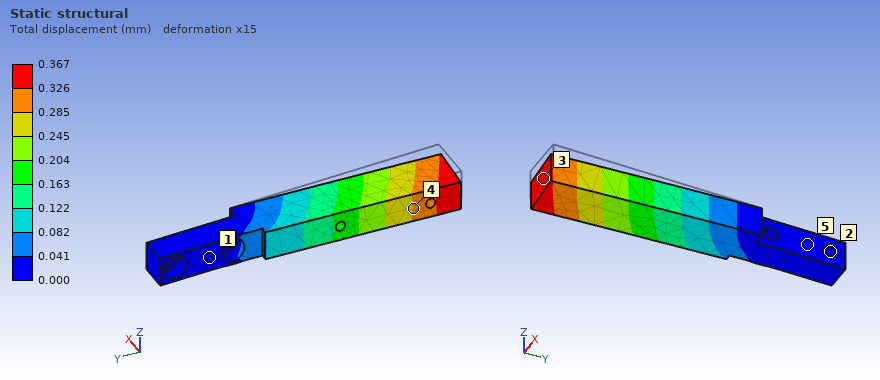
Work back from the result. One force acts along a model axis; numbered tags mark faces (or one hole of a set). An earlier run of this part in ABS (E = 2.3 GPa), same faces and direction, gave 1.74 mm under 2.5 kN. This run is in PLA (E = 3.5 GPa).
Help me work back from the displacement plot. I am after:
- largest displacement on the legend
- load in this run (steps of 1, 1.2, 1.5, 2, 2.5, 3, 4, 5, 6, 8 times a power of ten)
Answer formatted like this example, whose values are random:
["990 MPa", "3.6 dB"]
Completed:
["0.367 mm", "800 N"]
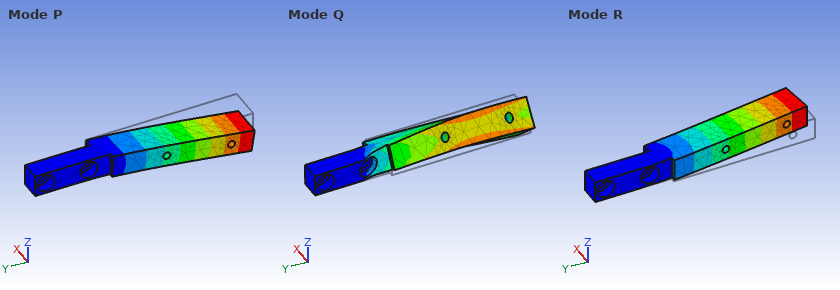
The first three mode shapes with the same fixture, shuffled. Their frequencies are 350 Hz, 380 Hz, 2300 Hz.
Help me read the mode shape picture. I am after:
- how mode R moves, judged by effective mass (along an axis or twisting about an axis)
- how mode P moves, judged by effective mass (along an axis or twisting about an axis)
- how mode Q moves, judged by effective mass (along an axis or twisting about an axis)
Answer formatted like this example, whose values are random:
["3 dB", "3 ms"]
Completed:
["along X", "along Z", "twisting about Y"]
